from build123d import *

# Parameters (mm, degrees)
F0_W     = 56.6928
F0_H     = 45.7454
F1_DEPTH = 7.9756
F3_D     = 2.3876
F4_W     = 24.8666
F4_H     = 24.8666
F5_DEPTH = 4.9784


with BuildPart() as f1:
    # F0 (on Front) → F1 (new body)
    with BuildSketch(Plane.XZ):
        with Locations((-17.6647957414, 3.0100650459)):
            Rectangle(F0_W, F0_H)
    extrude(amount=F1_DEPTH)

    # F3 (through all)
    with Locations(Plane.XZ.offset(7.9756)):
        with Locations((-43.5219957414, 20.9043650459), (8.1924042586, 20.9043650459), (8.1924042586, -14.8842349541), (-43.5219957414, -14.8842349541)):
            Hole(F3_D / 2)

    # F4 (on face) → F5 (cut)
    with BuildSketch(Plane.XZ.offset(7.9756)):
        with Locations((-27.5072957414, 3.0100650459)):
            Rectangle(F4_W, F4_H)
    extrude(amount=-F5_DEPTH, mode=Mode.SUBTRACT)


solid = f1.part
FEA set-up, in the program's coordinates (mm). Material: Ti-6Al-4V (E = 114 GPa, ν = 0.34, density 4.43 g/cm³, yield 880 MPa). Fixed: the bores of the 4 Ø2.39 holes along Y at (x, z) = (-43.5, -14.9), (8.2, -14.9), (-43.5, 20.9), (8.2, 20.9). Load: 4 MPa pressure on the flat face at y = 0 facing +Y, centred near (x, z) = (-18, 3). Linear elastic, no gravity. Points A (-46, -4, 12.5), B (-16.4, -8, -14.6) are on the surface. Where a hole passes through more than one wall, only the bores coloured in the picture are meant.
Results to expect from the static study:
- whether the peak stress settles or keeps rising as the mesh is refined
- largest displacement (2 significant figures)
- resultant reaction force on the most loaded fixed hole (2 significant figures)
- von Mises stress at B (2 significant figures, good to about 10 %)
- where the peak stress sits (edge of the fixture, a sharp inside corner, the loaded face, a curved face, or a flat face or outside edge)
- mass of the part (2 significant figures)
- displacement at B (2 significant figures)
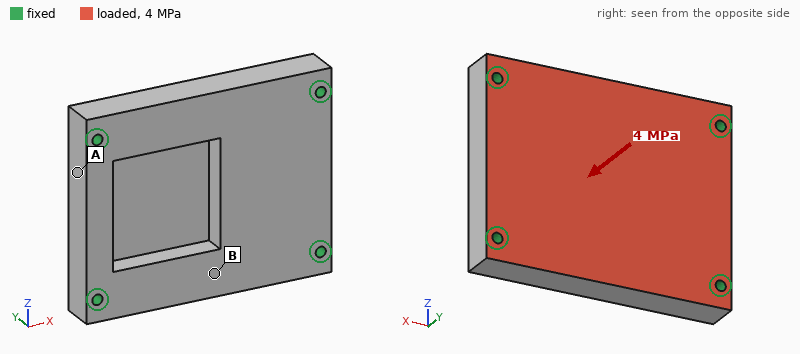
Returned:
keeps rising
60 µm
2.7 kN
82 MPa
edge of the fixture
77 g
40 µm
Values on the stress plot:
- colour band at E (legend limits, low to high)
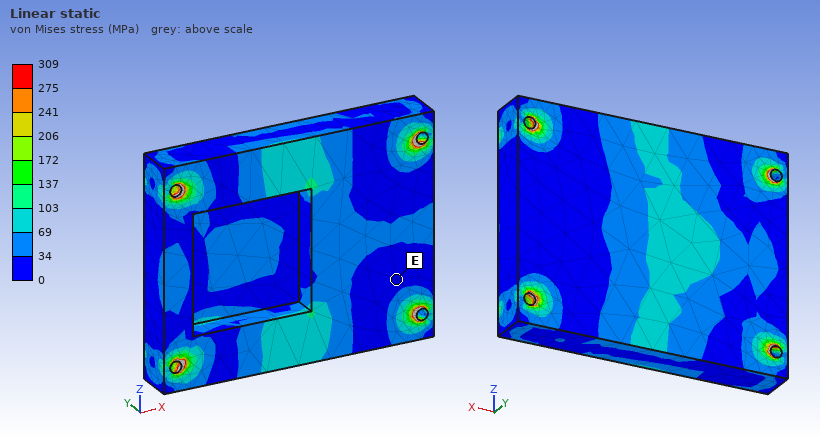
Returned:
0 to 34 MPa
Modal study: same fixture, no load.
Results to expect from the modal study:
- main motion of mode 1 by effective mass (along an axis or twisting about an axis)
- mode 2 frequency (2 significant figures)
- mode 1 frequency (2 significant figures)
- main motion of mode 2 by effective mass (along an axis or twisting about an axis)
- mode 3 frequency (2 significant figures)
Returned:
along Y
14 kHz
10 kHz
twisting about X
21 kHz
